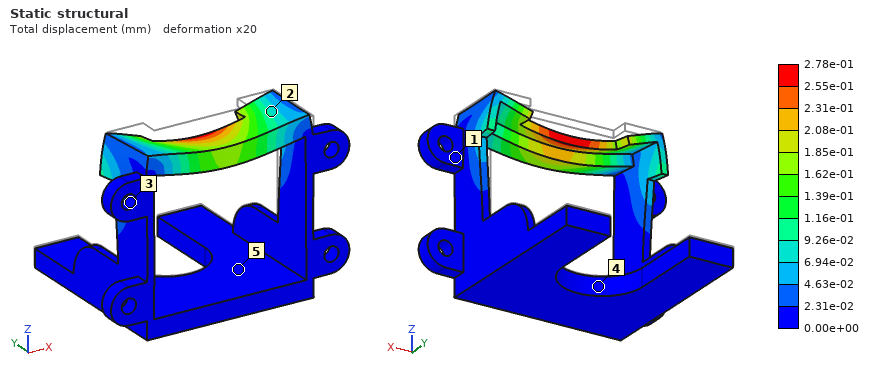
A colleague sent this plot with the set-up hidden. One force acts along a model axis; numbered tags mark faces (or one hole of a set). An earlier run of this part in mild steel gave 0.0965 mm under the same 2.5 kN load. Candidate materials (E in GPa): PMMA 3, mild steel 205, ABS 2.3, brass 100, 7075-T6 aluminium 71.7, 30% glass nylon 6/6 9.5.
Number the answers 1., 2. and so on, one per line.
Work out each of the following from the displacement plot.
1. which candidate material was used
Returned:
1. 7075-T6 aluminium
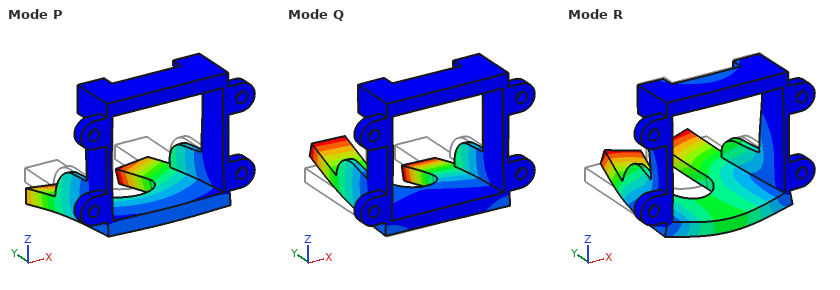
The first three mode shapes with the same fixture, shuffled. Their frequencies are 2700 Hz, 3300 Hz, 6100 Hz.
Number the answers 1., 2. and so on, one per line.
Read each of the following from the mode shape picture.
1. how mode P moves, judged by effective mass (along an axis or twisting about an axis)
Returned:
1. along Z
